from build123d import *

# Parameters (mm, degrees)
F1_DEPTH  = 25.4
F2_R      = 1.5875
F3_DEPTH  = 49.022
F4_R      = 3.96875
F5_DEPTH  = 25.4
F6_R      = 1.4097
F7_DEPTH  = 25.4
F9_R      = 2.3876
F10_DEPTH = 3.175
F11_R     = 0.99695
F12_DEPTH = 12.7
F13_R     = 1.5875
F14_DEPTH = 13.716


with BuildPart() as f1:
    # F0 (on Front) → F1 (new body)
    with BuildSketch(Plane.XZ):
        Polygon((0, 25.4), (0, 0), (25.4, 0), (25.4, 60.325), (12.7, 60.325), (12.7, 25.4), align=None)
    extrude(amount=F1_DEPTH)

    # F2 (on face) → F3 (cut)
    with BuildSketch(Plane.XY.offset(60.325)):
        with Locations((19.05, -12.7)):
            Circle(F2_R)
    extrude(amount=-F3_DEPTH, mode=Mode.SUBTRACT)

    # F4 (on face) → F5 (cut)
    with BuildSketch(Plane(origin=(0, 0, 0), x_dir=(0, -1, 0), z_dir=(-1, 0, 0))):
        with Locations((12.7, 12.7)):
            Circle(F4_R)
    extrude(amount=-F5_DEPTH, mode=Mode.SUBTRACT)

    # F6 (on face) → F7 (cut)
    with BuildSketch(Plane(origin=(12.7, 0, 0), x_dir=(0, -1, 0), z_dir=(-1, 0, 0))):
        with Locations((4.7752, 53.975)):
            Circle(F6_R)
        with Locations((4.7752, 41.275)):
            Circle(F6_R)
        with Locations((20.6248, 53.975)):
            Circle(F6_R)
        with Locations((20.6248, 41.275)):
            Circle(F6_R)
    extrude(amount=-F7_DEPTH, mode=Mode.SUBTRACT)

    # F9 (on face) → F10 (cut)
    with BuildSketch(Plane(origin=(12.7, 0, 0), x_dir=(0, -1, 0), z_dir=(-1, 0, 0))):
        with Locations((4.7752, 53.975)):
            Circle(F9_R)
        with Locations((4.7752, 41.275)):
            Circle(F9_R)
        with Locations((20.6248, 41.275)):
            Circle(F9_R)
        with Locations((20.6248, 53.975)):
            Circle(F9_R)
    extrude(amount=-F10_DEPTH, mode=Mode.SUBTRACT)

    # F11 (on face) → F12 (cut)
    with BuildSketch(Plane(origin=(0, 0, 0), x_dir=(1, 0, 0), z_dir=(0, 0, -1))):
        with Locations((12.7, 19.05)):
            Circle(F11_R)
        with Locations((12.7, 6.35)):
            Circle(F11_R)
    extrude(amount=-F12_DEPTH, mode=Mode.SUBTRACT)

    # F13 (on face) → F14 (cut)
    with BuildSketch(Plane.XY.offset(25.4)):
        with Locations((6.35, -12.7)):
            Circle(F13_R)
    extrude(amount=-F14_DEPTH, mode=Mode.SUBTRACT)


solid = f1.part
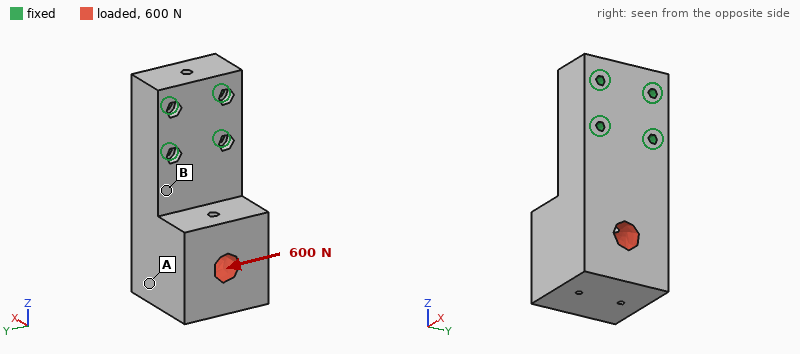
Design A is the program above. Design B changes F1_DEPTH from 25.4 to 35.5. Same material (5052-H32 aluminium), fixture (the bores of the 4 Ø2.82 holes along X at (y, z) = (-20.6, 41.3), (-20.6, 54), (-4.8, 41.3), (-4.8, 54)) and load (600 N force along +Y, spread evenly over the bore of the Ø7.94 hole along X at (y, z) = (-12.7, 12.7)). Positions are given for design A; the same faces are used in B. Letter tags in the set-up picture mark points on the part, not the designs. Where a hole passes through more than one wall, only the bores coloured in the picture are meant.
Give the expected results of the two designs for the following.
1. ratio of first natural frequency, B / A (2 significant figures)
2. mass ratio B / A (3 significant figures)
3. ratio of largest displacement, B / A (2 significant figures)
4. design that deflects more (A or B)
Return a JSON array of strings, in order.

["0.95", "1.43", "0.67", "A"]
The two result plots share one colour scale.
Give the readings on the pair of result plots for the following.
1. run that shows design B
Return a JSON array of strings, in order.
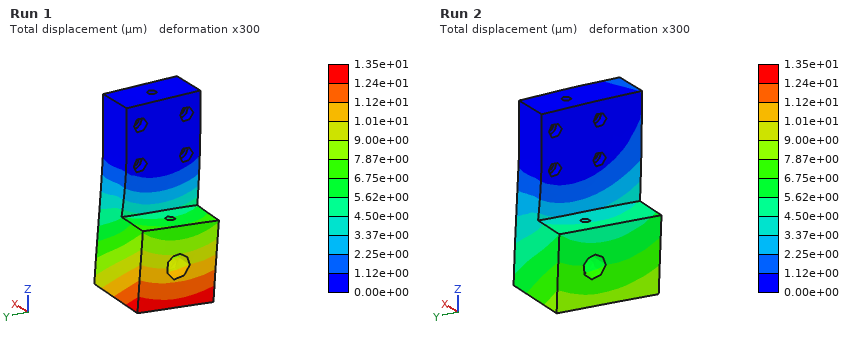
["Run 2"]
